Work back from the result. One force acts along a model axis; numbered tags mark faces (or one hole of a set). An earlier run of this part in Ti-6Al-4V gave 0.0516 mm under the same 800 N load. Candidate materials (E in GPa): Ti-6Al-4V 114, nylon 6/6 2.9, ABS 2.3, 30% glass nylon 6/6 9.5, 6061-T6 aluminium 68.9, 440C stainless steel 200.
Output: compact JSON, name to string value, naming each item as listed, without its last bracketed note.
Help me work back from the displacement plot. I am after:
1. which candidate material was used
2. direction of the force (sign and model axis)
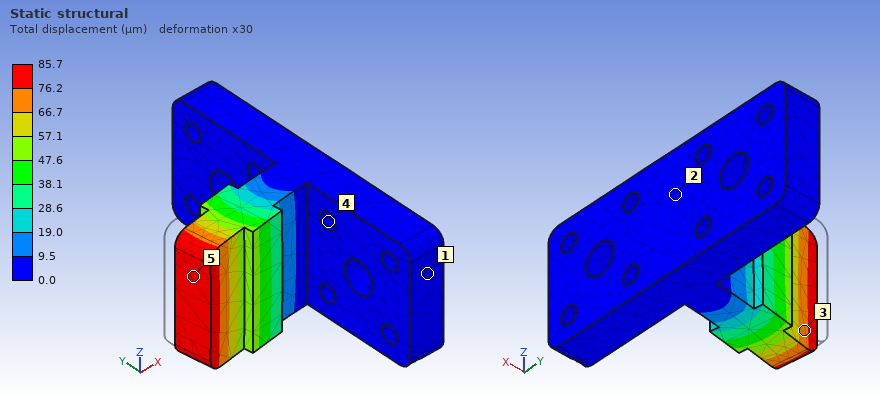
{"which candidate material was used": "6061-T6 aluminium", "direction of the force": "-Y"}
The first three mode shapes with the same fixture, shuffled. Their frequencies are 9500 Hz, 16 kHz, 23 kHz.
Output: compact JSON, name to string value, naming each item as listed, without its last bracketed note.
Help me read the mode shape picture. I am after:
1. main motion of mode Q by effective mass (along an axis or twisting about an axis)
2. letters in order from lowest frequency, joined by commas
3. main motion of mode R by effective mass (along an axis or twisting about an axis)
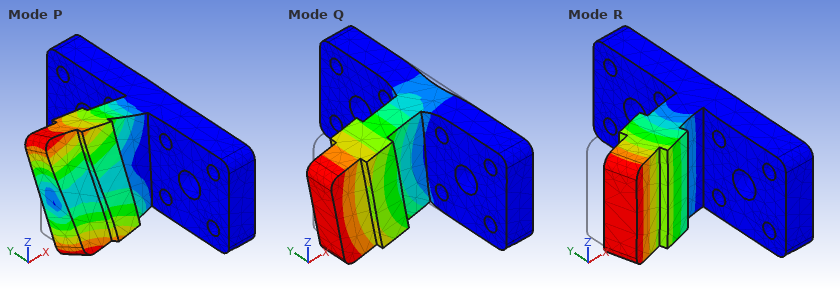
{"main motion of mode Q by effective mass": "along Z", "letters in order from lowest frequency, joined by commas": "R, Q, P", "main motion of mode R by effective mass": "along Y"}
